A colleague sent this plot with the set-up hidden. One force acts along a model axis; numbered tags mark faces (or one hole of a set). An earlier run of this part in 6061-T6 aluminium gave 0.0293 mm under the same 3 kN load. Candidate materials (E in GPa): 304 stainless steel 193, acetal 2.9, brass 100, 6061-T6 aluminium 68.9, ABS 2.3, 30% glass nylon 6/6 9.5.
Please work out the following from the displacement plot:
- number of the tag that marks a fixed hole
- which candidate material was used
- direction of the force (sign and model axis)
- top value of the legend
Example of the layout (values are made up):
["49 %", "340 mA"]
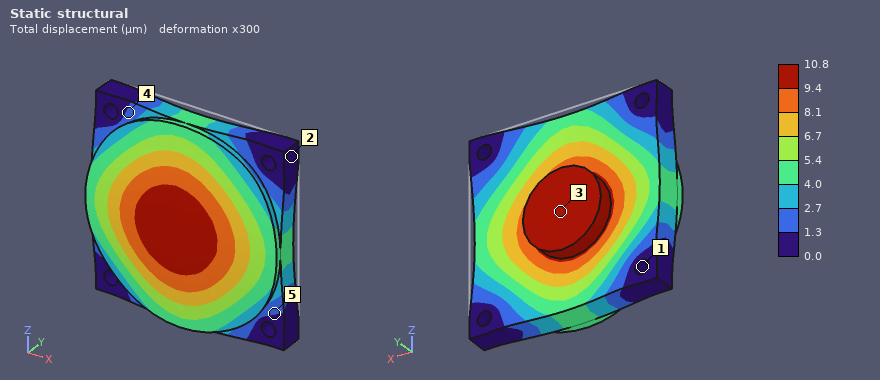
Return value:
["1", "304 stainless steel", "-Y", "10.8 µm"]
